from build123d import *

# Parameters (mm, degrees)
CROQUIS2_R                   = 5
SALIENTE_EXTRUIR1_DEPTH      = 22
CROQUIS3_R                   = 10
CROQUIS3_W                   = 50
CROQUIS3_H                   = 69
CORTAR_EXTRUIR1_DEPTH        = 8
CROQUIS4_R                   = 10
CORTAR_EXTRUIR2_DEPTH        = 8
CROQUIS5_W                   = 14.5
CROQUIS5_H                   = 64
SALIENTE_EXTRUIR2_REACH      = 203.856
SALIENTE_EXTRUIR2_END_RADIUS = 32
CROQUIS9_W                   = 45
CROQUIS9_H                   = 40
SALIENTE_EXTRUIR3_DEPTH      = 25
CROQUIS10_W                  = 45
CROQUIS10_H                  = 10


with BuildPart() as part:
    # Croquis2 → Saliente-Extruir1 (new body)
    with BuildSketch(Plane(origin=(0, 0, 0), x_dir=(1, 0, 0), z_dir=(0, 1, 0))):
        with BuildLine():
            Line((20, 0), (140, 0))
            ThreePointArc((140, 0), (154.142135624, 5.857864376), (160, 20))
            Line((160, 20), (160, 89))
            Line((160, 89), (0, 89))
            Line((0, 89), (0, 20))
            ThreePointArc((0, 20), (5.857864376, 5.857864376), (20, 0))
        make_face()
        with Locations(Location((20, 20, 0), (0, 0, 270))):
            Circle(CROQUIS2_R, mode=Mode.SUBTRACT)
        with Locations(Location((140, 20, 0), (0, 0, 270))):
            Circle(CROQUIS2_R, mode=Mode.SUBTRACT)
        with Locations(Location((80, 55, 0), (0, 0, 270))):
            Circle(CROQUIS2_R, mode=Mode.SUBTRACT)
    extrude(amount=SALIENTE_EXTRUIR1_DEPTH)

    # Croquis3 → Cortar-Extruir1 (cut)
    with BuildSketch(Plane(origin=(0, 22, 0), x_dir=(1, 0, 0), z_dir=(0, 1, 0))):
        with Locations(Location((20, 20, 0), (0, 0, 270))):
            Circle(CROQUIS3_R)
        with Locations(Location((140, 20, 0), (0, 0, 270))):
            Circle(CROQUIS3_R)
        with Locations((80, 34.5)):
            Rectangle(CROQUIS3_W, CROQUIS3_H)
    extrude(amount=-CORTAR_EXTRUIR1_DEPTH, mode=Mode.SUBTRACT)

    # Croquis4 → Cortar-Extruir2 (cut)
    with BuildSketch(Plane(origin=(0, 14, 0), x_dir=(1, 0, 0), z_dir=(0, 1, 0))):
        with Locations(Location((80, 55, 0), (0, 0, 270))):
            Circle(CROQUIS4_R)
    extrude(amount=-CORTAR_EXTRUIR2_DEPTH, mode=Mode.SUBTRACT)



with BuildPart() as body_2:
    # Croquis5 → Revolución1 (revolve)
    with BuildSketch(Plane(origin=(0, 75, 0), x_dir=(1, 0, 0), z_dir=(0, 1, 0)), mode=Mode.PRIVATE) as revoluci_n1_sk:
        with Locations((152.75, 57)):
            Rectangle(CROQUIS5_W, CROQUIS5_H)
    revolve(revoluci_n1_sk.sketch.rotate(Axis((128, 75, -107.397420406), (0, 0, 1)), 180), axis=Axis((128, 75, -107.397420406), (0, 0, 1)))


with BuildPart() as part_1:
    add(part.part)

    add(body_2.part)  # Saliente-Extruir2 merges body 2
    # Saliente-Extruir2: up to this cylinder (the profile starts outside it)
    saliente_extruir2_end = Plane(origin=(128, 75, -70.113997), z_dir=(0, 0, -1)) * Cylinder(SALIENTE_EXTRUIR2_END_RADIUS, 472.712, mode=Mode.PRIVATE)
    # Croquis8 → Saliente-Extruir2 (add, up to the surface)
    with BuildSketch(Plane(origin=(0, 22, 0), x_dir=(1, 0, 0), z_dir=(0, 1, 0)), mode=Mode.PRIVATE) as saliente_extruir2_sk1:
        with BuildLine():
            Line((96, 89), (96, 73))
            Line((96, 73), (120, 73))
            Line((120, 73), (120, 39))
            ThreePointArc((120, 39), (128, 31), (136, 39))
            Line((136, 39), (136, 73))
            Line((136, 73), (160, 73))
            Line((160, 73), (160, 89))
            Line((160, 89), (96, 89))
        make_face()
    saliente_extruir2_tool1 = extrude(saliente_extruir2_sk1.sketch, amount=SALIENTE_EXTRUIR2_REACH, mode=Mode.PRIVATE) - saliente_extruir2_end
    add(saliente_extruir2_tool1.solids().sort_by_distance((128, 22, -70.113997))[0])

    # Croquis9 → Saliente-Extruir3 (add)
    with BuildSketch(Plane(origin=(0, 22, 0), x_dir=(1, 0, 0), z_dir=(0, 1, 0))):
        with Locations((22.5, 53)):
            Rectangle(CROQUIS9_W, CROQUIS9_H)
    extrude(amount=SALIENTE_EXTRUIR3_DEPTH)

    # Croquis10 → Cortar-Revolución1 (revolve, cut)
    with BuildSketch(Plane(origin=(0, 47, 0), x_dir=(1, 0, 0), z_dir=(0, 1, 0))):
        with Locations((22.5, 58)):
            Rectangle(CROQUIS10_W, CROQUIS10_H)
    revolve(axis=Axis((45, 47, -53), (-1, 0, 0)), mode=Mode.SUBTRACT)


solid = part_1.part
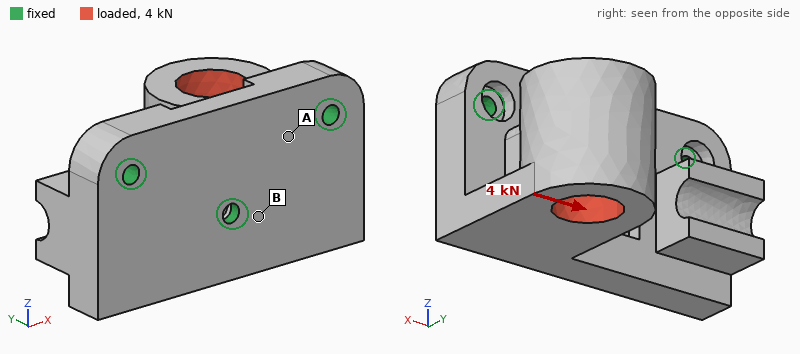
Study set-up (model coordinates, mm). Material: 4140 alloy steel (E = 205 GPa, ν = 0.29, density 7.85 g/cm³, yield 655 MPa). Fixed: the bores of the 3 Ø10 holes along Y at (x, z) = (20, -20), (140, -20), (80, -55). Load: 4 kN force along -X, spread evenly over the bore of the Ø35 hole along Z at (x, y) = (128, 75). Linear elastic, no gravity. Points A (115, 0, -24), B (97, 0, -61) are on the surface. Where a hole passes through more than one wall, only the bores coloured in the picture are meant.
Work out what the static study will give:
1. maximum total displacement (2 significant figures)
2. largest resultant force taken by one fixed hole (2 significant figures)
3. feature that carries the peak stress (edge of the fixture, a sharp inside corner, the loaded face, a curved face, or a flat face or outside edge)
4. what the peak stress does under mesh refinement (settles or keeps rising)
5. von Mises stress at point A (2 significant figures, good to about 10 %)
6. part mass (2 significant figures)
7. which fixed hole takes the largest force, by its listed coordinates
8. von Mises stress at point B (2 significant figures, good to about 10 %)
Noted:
67 µm
3.8 kN
edge of the fixture
keeps rising
9.7 MPa
3.9 kg
(140, -20)
19 MPa
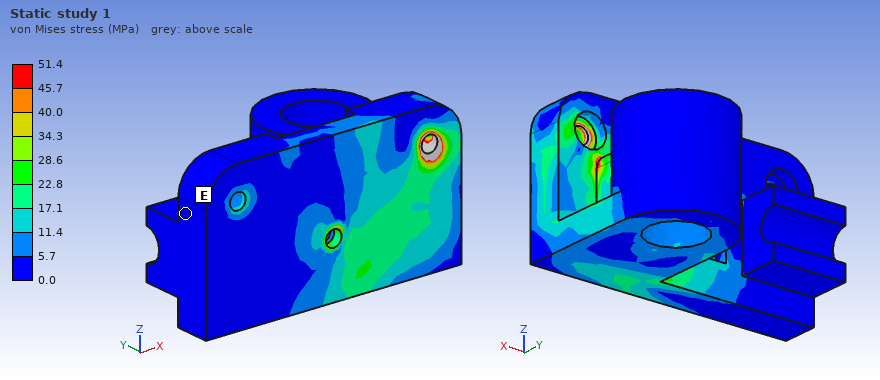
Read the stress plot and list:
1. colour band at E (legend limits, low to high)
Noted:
0.0 to 5.7 MPa
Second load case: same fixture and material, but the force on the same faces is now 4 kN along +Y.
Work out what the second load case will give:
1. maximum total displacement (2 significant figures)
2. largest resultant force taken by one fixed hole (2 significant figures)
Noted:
28 µm
2.5 kN
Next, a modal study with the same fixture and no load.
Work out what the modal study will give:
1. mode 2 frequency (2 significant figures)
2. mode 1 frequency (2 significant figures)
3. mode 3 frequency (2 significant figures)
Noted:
1800 Hz
990 Hz
3000 Hz
